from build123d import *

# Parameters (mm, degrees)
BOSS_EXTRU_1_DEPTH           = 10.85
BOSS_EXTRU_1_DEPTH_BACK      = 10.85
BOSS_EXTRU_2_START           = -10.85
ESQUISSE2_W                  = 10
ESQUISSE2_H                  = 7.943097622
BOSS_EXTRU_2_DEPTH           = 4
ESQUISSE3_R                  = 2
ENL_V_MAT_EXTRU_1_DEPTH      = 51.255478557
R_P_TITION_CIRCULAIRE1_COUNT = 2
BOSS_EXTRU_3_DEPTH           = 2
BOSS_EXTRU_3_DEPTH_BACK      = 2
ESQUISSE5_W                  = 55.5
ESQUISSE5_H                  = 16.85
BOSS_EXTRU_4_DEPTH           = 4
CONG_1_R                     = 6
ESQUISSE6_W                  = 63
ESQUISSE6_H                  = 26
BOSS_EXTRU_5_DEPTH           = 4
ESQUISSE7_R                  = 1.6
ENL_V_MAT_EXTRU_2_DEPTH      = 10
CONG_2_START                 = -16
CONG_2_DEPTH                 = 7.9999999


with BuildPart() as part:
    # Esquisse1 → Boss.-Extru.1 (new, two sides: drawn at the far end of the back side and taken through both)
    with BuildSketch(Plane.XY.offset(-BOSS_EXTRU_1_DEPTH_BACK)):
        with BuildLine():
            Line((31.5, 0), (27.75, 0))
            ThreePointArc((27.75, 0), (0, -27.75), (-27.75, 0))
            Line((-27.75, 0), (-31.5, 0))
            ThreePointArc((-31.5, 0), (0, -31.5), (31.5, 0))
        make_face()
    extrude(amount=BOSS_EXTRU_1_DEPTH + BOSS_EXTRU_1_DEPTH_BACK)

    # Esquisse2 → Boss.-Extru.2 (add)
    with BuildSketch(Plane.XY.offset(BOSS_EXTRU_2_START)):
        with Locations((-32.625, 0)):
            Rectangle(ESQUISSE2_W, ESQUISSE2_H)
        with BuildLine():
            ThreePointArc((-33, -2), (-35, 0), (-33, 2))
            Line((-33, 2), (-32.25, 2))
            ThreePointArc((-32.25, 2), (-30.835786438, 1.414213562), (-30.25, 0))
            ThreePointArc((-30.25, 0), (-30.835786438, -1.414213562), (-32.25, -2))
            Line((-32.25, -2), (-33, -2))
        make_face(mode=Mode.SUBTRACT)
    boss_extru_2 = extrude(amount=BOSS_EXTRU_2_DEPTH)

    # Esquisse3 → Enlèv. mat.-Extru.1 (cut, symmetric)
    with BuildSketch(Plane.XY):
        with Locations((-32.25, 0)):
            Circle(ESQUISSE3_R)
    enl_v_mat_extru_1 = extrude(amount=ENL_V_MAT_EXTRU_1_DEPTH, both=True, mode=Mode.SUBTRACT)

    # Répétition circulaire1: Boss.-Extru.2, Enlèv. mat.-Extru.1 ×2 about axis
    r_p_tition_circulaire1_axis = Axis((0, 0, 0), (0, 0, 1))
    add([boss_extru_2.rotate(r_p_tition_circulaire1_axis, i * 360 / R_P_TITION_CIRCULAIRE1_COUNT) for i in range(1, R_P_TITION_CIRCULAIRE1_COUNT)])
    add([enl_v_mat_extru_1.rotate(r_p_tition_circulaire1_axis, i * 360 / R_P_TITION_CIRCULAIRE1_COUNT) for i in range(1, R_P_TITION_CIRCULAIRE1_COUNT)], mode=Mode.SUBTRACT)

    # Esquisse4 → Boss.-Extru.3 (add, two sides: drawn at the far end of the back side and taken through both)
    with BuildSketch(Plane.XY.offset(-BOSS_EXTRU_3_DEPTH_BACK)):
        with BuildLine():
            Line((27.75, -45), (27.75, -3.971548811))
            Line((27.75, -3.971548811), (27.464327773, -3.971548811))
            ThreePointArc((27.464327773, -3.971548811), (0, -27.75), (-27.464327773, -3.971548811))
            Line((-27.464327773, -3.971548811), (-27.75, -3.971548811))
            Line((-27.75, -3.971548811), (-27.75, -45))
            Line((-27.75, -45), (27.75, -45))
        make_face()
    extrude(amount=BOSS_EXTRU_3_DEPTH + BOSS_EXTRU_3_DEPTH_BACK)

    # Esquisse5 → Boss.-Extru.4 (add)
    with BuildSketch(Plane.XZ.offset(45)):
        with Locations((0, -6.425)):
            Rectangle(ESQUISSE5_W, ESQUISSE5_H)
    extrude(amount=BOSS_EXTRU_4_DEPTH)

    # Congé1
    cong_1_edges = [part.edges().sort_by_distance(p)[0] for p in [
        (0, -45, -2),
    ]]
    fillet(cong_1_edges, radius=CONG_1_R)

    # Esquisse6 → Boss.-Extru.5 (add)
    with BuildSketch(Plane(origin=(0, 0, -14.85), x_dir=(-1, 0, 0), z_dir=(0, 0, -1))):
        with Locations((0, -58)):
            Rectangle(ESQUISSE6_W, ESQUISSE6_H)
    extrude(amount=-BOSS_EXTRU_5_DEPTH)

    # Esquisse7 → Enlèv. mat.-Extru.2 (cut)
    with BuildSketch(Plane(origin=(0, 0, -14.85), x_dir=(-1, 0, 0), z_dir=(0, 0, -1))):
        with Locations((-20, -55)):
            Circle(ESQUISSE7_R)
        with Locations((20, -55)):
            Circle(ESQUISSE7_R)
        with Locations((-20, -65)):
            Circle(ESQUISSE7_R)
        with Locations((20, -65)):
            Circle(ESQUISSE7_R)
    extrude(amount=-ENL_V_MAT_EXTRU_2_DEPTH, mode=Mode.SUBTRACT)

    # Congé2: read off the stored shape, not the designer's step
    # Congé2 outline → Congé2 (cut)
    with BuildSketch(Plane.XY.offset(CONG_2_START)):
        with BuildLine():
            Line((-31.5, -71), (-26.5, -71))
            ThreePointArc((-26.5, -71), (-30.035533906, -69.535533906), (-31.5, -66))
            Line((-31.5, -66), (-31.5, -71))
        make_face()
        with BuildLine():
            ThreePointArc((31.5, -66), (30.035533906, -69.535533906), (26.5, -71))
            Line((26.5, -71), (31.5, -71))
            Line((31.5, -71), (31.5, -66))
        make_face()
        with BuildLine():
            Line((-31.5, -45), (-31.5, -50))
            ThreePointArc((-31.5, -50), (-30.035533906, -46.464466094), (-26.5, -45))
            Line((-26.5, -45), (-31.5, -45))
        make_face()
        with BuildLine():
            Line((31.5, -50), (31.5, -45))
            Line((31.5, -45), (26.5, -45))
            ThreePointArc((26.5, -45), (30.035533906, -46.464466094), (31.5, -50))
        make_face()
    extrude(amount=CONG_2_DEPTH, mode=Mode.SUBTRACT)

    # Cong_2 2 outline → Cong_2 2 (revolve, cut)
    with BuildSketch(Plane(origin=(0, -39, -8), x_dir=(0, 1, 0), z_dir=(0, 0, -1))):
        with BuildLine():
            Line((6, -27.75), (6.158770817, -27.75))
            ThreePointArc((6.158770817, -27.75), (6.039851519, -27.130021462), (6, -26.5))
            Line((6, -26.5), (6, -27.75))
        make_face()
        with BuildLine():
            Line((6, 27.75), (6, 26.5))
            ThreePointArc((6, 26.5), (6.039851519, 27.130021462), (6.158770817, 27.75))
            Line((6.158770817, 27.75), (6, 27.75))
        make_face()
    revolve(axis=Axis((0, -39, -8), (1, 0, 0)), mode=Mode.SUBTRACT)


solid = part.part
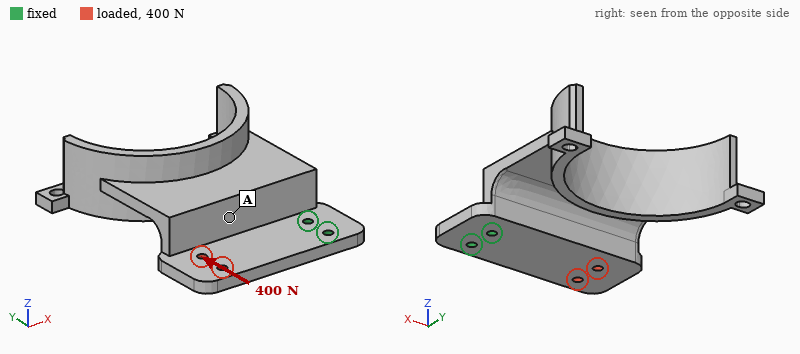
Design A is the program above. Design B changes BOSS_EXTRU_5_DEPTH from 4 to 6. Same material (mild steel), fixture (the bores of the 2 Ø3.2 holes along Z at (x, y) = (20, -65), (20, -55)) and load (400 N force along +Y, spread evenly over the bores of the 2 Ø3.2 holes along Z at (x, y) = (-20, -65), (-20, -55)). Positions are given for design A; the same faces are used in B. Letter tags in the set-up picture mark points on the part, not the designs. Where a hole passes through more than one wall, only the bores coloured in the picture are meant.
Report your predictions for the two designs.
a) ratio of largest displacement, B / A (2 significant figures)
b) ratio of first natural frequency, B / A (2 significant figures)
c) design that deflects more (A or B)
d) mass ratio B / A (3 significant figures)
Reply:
0.68
1.4
A
1.13
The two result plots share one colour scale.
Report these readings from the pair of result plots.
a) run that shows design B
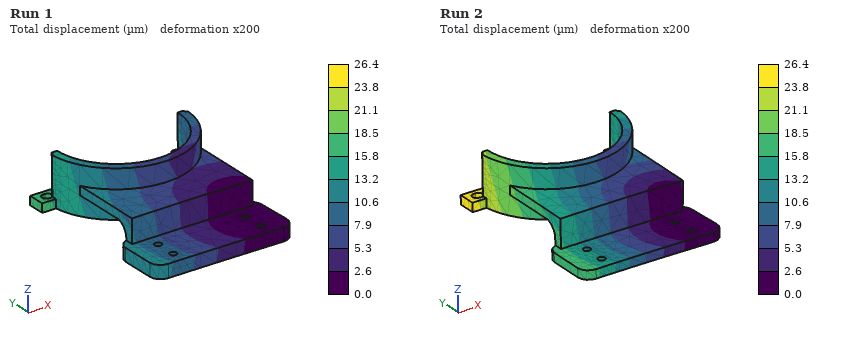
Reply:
Run 1
